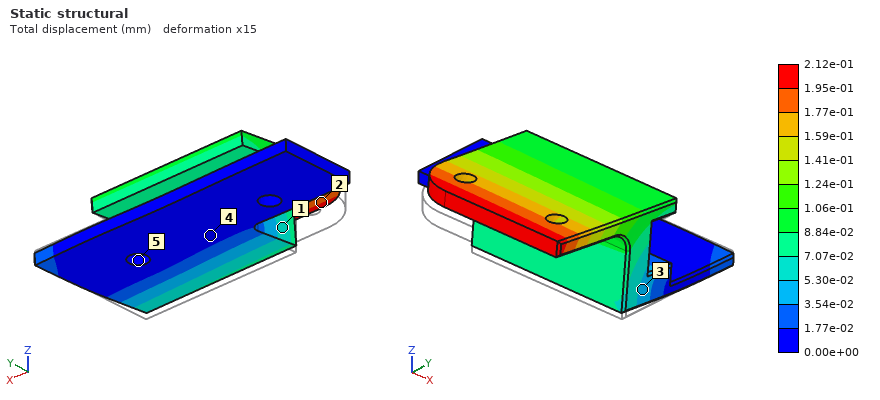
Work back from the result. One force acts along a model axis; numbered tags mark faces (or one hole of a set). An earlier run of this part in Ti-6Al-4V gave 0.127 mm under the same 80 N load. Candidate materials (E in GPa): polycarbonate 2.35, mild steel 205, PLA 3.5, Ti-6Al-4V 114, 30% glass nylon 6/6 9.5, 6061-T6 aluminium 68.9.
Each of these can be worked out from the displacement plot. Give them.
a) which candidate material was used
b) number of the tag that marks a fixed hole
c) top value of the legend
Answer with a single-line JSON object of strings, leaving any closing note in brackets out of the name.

{"which candidate material was used": "6061-T6 aluminium", "number of the tag that marks a fixed hole": "5", "top value of the legend": "2.12e-01 mm"}
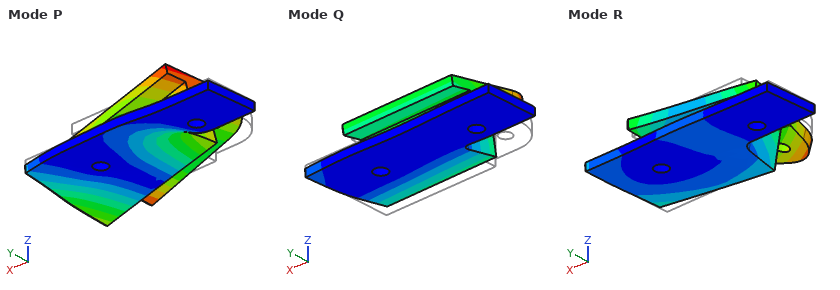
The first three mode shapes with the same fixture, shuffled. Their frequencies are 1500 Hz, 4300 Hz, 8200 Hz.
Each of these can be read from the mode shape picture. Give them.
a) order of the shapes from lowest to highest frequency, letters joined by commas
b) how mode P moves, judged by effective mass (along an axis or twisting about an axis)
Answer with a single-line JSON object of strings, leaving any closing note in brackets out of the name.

{"order of the shapes from lowest to highest frequency, letters joined by commas": "Q, P, R", "how mode P moves, judged by effective mass": "along X"}
